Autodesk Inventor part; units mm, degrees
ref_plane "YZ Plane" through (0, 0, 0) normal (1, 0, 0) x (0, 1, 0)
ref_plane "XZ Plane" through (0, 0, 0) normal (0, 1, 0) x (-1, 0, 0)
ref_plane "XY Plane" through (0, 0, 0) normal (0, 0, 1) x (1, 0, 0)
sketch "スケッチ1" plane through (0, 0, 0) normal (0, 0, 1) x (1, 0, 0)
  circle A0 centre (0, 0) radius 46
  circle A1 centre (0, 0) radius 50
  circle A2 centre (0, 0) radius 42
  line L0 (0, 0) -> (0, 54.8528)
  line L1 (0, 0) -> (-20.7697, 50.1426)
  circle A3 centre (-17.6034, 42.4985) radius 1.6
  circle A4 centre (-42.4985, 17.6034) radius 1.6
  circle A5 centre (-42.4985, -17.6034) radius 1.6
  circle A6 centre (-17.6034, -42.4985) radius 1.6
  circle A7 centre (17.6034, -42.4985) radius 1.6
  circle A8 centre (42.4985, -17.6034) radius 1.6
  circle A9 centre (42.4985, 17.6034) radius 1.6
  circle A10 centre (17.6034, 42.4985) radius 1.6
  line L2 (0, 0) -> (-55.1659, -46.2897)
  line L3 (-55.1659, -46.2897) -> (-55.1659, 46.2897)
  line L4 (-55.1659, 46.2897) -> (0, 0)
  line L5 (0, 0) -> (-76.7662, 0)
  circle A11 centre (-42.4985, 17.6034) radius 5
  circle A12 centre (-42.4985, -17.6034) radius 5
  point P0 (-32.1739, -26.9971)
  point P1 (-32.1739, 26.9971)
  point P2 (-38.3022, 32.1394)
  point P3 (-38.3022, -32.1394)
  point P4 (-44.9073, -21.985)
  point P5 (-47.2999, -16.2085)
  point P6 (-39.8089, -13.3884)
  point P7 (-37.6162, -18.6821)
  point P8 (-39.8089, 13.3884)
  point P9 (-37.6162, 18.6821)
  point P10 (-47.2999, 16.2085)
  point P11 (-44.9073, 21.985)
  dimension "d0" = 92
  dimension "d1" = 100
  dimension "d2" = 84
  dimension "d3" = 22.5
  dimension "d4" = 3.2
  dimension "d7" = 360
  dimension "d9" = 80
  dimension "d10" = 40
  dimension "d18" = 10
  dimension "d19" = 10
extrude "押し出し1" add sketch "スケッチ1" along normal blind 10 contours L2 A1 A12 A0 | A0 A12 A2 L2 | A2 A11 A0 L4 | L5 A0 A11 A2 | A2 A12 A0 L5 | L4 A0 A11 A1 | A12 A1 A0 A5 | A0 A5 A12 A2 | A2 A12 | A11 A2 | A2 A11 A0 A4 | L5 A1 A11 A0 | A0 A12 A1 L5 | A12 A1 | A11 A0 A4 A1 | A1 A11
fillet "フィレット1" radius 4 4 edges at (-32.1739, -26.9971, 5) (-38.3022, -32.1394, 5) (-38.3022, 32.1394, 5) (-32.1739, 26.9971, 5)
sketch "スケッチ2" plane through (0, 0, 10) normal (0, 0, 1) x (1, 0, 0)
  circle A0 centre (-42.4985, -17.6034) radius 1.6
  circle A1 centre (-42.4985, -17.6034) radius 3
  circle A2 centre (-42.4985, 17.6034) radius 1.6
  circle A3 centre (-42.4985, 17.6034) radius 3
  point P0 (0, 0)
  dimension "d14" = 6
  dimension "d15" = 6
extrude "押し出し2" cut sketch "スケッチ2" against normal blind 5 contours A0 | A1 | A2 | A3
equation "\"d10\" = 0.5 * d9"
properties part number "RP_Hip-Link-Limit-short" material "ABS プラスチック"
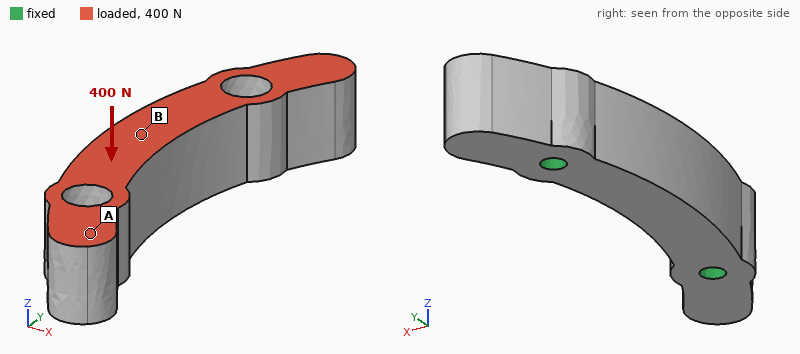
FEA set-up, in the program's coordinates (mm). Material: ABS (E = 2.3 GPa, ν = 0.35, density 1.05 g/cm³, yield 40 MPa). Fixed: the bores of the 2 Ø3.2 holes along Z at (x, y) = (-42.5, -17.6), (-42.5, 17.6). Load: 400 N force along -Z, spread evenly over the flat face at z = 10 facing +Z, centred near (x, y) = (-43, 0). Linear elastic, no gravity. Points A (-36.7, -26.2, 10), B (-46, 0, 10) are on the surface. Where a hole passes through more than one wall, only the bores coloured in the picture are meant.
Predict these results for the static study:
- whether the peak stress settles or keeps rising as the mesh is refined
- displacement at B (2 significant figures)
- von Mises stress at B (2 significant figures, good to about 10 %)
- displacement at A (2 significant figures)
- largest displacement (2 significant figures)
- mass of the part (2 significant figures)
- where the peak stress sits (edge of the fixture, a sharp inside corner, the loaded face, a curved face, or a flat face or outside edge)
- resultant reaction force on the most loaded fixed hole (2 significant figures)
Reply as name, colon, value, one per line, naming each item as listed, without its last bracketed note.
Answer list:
whether the peak stress settles or keeps rising as the mesh is refined: keeps rising
displacement at B: 52 µm
von Mises stress at B: 3.2 MPa
displacement at A: 34 µm
largest displacement: 62 µm
mass of the part: 5.0 g
where the peak stress sits: edge of the fixture
resultant reaction force on the most loaded fixed hole: 200 N
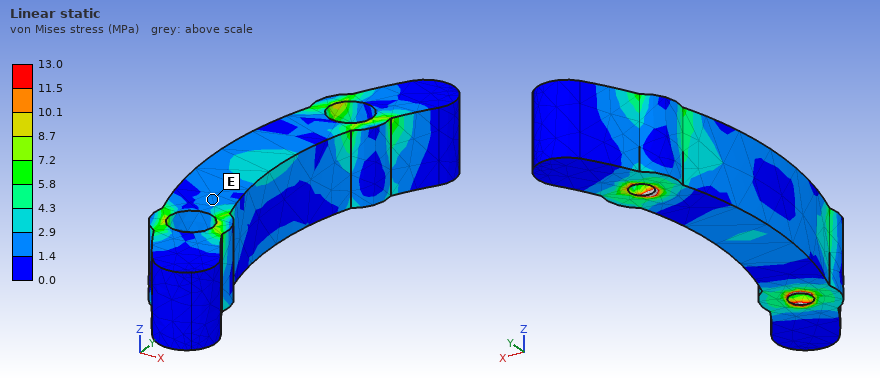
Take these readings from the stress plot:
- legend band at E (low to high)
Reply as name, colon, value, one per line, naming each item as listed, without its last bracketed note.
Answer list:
legend band at E: 1.4 to 2.9 MPa
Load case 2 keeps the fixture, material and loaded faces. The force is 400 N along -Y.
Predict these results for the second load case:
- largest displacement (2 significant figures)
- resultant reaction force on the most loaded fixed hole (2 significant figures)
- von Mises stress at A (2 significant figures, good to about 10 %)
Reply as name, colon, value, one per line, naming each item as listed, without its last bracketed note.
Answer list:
largest displacement: 93 µm
resultant reaction force on the most loaded fixed hole: 210 N
von Mises stress at A: 2.3 MPa
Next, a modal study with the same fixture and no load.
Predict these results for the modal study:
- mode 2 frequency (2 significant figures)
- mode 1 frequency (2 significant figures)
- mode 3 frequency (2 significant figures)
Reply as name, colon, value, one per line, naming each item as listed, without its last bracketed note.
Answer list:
mode 2 frequency: 6100 Hz
mode 1 frequency: 5000 Hz
mode 3 frequency: 6600 Hz
